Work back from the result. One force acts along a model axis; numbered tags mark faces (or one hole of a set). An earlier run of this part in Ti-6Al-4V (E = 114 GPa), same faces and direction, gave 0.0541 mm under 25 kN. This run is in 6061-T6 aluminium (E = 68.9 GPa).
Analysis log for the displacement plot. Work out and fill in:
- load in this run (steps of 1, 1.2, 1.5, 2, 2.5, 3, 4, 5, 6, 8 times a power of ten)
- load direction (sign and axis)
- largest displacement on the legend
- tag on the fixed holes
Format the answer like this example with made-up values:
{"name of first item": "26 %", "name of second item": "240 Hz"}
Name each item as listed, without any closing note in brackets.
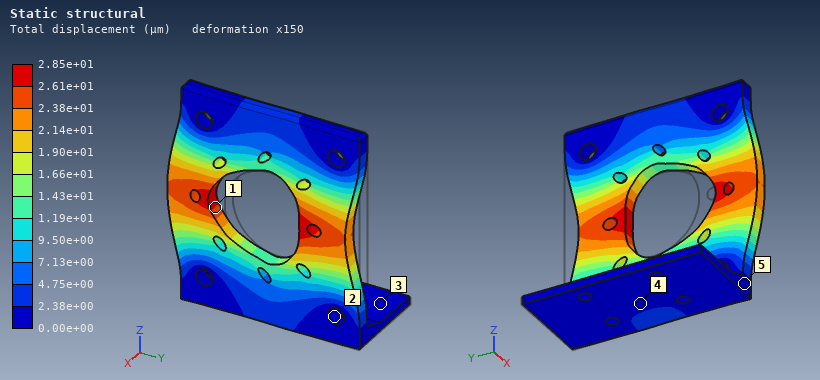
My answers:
{"load in this run": "8 kN", "load direction": "-Y", "largest displacement on the legend": "2.85e+01 µm", "tag on the fixed holes": "2"}
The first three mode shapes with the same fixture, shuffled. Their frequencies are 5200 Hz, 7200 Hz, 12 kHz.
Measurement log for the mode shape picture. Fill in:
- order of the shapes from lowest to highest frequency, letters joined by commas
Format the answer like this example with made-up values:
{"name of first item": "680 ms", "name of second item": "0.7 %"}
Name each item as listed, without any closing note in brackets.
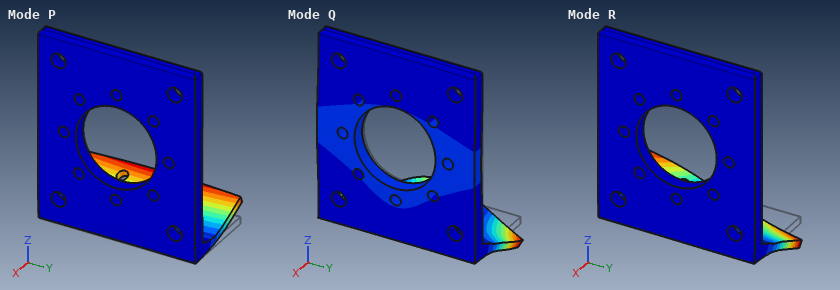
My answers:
{"order of the shapes from lowest to highest frequency, letters joined by commas": "P, R, Q"}
